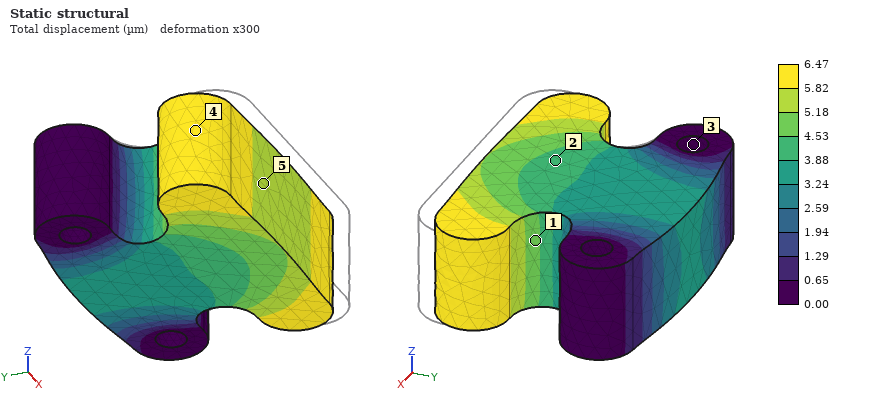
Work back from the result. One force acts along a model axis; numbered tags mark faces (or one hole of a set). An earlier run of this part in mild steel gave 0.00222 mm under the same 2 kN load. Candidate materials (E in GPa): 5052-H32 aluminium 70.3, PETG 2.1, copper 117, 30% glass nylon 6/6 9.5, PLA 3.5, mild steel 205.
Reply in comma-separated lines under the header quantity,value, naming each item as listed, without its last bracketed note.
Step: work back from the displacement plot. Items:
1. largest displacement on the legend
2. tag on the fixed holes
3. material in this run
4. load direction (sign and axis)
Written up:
quantity,value
largest displacement on the legend,6.47 µm
tag on the fixed holes,3
material in this run,5052-H32 aluminium
load direction,+Y
